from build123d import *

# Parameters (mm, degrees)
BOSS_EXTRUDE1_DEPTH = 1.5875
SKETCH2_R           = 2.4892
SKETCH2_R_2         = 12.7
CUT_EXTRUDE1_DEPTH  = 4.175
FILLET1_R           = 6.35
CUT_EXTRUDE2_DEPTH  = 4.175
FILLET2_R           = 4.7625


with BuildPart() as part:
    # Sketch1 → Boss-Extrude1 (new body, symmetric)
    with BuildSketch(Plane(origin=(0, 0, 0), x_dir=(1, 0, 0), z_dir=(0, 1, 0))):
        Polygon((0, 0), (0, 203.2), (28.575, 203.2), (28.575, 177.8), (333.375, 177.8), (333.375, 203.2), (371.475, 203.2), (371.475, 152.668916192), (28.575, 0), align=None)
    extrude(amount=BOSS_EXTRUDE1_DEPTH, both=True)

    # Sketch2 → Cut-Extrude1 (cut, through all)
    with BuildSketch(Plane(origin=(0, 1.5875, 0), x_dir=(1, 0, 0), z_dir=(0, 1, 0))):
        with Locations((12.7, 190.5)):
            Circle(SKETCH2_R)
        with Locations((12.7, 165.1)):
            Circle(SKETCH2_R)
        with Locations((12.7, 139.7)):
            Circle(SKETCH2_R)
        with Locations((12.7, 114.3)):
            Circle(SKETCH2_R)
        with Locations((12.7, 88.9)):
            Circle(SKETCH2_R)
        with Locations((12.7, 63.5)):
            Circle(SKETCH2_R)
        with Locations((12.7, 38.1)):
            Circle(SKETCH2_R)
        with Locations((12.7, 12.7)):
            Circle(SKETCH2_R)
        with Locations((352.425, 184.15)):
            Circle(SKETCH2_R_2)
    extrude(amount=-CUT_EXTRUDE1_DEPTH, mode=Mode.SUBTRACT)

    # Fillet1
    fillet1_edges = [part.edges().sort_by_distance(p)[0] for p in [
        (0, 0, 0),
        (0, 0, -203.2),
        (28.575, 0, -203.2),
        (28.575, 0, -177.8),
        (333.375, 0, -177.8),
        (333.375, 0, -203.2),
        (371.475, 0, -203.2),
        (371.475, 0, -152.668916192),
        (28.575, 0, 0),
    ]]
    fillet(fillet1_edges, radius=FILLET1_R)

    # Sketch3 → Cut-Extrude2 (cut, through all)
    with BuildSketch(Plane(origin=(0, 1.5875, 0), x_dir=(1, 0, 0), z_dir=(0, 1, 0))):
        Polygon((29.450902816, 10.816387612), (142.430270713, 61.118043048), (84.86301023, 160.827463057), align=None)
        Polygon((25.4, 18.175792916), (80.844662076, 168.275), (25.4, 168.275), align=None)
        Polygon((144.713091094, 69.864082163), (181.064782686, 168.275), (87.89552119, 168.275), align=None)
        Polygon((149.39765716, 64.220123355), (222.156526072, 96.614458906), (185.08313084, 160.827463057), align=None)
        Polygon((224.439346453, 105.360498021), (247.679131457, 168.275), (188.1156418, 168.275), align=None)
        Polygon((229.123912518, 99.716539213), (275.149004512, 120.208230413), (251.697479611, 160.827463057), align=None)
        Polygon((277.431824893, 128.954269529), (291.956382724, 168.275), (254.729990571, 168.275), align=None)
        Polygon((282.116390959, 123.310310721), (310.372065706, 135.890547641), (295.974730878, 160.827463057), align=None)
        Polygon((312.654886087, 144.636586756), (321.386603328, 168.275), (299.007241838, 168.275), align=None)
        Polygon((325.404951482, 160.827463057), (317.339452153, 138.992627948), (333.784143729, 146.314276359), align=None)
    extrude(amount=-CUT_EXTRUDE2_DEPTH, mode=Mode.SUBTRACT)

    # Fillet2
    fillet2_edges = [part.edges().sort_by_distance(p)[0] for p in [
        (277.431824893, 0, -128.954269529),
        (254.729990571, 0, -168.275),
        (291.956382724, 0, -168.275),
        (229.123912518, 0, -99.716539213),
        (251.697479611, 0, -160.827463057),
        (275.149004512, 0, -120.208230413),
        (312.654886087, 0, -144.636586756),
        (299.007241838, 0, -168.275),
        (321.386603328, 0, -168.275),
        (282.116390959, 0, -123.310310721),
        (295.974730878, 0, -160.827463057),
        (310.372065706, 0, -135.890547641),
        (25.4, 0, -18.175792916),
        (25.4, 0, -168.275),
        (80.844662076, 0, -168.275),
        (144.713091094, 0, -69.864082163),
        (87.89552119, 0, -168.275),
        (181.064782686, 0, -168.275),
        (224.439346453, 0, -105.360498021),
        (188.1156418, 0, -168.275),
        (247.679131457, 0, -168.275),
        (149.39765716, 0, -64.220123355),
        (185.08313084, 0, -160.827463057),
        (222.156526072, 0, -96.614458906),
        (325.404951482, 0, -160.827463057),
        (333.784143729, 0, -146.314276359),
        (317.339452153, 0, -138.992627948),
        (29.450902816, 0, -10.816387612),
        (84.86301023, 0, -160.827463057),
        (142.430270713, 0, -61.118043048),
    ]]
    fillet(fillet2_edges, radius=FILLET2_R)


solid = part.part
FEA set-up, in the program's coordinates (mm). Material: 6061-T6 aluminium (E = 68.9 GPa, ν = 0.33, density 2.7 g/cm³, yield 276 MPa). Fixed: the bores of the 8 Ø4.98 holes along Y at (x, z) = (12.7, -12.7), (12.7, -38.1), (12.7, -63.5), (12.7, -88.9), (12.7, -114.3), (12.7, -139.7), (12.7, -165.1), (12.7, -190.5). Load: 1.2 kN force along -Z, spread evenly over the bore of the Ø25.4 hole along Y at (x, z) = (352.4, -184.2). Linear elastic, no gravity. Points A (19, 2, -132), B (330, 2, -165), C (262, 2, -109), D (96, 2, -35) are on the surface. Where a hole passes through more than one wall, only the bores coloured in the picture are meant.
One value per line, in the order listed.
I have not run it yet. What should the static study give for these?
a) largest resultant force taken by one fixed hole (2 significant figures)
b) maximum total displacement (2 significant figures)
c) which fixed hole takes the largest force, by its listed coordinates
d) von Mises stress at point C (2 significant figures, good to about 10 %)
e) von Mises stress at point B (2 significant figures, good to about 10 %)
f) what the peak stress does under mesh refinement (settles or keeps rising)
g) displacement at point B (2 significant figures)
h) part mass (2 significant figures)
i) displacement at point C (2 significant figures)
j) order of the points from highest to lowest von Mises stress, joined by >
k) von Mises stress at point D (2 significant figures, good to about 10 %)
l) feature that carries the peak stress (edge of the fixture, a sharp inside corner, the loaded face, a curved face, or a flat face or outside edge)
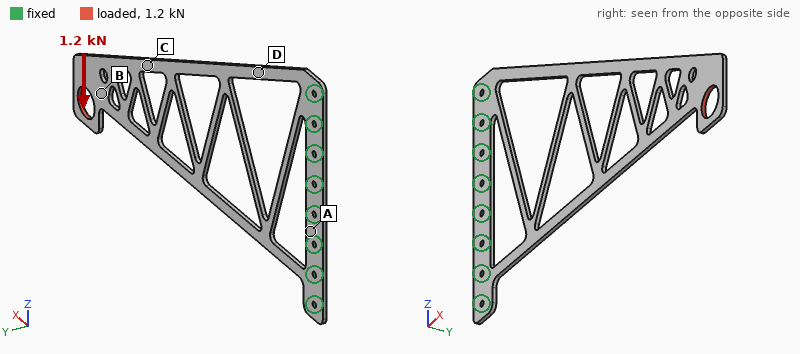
3.2 kN
1.4 mm
(12.7, -12.7)
64 MPa
23 MPa
keeps rising
1.1 mm
150 g
0.64 mm
D > C > B > A
81 MPa
edge of the fixture
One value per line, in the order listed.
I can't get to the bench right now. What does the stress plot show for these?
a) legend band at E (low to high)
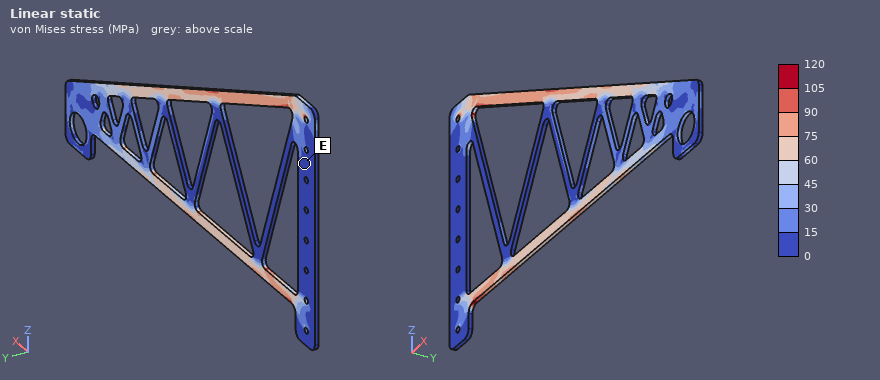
0 to 15 MPa
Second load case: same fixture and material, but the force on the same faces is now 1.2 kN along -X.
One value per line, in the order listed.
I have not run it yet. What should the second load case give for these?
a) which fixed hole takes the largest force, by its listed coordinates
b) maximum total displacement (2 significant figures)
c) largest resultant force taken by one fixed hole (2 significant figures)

(12.7, -165.1)
0.55 mm
830 N
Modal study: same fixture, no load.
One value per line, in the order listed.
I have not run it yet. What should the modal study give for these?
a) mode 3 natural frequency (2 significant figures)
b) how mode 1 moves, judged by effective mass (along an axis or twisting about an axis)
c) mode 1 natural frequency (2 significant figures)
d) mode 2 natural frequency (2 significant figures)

150 Hz
along Y
16 Hz
97 Hz
